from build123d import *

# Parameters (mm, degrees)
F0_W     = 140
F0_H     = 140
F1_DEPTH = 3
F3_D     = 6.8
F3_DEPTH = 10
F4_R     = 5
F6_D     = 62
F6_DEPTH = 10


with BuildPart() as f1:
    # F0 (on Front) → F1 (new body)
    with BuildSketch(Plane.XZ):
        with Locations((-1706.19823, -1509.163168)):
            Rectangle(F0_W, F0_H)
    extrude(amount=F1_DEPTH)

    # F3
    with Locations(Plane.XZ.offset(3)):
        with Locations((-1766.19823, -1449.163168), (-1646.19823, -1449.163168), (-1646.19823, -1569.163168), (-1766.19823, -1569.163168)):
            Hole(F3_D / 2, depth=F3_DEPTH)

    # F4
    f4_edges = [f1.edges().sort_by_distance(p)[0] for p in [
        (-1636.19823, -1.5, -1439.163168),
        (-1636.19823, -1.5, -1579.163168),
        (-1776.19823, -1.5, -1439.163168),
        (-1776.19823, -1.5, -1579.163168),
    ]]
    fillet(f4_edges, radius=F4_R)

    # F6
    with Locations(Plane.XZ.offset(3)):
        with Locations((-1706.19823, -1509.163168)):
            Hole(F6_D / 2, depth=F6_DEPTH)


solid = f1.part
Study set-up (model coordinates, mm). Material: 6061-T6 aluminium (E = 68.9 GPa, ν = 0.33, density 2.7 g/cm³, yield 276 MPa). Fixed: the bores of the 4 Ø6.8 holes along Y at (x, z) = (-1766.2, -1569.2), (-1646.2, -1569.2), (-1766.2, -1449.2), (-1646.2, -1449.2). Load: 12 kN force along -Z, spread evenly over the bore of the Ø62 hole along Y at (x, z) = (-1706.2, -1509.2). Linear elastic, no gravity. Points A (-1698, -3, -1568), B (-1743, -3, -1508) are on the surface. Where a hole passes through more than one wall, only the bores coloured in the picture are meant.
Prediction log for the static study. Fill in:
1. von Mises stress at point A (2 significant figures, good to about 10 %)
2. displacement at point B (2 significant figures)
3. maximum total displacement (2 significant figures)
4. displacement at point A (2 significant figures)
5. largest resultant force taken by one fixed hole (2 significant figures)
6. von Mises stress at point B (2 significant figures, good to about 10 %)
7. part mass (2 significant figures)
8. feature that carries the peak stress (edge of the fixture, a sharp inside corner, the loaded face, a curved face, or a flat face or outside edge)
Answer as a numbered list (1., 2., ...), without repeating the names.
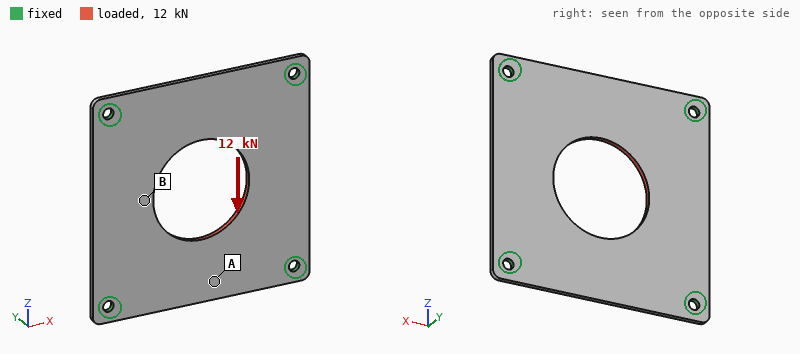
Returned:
1. 14 MPa
2. 28 µm
3. 48 µm
4. 42 µm
5. 3.3 kN
6. 38 MPa
7. 130 g
8. edge of the fixture
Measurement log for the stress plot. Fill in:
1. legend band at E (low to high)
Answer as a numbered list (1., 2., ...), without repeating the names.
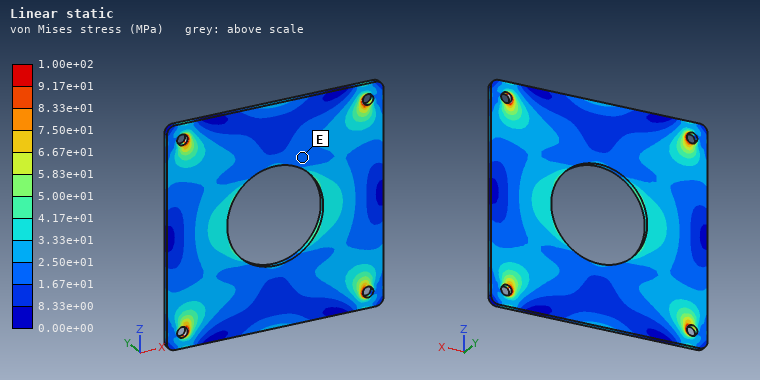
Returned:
1. 1.67e+01 to 2.50e+01 MPa
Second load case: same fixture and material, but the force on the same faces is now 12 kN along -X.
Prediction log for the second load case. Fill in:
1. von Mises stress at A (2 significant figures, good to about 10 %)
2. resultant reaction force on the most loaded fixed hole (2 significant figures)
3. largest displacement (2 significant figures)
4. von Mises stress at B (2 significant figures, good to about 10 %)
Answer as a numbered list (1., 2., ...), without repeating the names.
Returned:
1. 17 MPa
2. 3.3 kN
3. 48 µm
4. 18 MPa
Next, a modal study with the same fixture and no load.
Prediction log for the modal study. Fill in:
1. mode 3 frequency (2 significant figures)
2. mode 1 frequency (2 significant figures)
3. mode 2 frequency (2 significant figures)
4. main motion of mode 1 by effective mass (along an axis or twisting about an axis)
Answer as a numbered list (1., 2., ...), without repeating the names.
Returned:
1. 1200 Hz
2. 810 Hz
3. 1200 Hz
4. along Y
